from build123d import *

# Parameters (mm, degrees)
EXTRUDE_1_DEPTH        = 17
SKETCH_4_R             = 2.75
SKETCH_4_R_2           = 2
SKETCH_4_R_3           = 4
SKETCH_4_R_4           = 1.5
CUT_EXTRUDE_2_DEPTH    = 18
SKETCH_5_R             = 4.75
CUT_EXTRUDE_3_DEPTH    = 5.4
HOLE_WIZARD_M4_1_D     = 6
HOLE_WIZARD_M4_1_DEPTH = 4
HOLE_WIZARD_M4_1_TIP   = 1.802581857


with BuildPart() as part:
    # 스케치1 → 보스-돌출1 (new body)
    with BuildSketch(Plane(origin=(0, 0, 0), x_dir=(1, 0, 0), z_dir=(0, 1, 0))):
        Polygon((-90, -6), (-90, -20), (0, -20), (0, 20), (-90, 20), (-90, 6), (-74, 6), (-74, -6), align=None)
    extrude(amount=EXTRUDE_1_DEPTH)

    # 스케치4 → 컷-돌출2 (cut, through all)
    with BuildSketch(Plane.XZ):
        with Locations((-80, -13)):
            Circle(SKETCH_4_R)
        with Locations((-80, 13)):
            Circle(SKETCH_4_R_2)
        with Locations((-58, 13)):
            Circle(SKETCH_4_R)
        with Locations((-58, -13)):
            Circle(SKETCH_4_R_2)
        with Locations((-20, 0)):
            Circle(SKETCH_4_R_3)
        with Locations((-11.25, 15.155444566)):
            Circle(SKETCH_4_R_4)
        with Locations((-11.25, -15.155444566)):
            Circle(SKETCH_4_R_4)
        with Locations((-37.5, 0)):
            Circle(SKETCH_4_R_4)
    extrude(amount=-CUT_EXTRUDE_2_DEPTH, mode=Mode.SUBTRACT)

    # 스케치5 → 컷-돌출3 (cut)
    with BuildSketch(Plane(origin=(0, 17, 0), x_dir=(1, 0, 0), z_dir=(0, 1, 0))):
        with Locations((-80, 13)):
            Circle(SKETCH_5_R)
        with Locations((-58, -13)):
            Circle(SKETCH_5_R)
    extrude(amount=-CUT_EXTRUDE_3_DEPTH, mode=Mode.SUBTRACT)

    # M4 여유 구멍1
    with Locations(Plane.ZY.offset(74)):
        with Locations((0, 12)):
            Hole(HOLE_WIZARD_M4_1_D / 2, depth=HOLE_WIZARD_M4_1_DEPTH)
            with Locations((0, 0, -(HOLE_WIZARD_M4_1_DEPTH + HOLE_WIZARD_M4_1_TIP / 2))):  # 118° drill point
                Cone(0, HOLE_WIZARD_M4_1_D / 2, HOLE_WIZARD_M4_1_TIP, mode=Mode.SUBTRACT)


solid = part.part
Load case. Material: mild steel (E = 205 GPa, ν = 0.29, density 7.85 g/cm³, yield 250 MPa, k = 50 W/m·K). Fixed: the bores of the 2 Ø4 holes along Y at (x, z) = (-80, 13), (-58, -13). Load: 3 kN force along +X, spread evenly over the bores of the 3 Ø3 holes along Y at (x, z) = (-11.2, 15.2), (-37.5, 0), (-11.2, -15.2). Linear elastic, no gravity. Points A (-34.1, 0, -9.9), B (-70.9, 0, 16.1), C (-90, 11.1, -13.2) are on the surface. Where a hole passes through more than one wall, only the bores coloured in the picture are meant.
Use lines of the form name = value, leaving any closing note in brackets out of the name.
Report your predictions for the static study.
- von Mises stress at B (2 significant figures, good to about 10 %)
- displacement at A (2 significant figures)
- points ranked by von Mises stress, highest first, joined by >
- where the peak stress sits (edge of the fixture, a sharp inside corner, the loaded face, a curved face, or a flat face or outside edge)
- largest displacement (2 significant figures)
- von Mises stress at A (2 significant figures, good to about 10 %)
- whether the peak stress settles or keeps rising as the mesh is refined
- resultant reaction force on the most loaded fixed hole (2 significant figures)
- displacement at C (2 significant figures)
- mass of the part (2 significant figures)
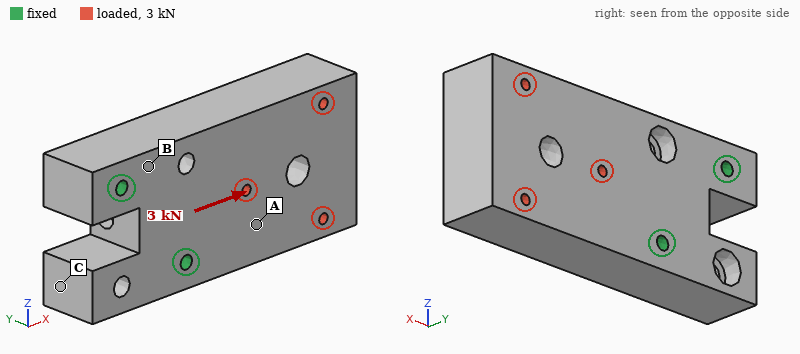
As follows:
von Mises stress at B = 6.7 MPa
displacement at A = 0.93 µm
points ranked by von Mises stress, highest first, joined by > = B > A > C
where the peak stress sits = edge of the fixture
largest displacement = 2.7 µm
von Mises stress at A = 3.6 MPa
whether the peak stress settles or keeps rising as the mesh is refined = keeps rising
resultant reaction force on the most loaded fixed hole = 1.5 kN
displacement at C = 0.74 µm
mass of the part = 430 g
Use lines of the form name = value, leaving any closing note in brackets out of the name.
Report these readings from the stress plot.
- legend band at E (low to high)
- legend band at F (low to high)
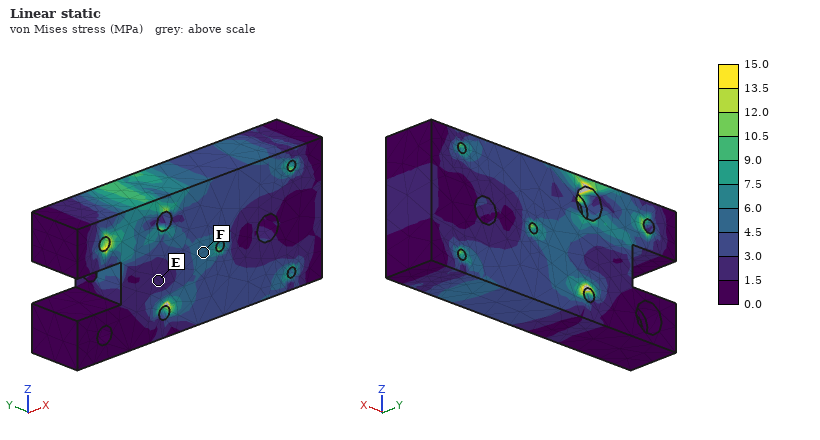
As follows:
legend band at E = 1.5 to 3.0 MPa
legend band at F = 4.5 to 6.0 MPa
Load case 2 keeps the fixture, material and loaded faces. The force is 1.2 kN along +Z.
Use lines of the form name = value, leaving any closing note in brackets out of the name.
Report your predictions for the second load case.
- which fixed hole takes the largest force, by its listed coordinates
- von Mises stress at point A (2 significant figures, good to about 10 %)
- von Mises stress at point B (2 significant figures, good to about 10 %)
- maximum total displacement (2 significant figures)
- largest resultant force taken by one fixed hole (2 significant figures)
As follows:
which fixed hole takes the largest force, by its listed coordinates = (-58, -13)
von Mises stress at point A = 3.0 MPa
von Mises stress at point B = 8.2 MPa
maximum total displacement = 6.2 µm
largest resultant force taken by one fixed hole = 2.0 kN
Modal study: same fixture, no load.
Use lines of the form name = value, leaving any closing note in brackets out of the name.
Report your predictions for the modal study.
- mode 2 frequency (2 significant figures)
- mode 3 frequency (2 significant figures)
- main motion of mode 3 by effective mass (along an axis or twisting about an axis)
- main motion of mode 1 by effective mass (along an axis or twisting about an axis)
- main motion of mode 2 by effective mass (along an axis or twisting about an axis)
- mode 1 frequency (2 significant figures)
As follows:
mode 2 frequency = 5700 Hz
mode 3 frequency = 8000 Hz
main motion of mode 3 by effective mass = twisting about X
main motion of mode 1 by effective mass = along Y
main motion of mode 2 by effective mass = along Z
mode 1 frequency = 3000 Hz
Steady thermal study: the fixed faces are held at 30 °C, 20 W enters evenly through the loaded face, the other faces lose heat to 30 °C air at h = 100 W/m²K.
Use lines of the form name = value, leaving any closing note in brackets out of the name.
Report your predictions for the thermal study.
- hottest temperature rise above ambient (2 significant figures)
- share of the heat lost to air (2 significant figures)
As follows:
hottest temperature rise above ambient = 18 K
share of the heat lost to air = 47 %
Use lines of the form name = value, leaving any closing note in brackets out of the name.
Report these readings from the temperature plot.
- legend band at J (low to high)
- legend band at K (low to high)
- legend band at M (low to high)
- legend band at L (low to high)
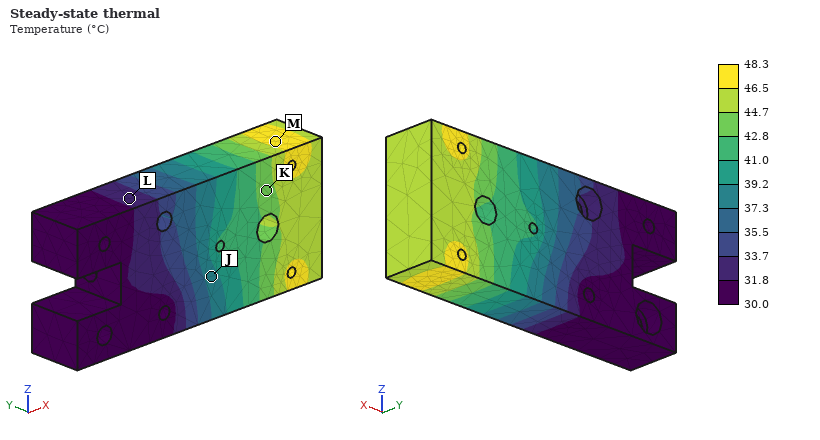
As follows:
legend band at J = 37.3 to 39.2 °C
legend band at K = 42.8 to 44.7 °C
legend band at M = 46.5 to 48.3 °C
legend band at L = 31.8 to 33.7 °C
